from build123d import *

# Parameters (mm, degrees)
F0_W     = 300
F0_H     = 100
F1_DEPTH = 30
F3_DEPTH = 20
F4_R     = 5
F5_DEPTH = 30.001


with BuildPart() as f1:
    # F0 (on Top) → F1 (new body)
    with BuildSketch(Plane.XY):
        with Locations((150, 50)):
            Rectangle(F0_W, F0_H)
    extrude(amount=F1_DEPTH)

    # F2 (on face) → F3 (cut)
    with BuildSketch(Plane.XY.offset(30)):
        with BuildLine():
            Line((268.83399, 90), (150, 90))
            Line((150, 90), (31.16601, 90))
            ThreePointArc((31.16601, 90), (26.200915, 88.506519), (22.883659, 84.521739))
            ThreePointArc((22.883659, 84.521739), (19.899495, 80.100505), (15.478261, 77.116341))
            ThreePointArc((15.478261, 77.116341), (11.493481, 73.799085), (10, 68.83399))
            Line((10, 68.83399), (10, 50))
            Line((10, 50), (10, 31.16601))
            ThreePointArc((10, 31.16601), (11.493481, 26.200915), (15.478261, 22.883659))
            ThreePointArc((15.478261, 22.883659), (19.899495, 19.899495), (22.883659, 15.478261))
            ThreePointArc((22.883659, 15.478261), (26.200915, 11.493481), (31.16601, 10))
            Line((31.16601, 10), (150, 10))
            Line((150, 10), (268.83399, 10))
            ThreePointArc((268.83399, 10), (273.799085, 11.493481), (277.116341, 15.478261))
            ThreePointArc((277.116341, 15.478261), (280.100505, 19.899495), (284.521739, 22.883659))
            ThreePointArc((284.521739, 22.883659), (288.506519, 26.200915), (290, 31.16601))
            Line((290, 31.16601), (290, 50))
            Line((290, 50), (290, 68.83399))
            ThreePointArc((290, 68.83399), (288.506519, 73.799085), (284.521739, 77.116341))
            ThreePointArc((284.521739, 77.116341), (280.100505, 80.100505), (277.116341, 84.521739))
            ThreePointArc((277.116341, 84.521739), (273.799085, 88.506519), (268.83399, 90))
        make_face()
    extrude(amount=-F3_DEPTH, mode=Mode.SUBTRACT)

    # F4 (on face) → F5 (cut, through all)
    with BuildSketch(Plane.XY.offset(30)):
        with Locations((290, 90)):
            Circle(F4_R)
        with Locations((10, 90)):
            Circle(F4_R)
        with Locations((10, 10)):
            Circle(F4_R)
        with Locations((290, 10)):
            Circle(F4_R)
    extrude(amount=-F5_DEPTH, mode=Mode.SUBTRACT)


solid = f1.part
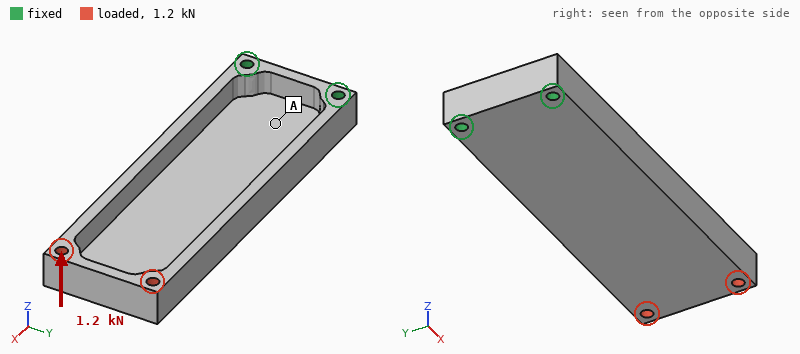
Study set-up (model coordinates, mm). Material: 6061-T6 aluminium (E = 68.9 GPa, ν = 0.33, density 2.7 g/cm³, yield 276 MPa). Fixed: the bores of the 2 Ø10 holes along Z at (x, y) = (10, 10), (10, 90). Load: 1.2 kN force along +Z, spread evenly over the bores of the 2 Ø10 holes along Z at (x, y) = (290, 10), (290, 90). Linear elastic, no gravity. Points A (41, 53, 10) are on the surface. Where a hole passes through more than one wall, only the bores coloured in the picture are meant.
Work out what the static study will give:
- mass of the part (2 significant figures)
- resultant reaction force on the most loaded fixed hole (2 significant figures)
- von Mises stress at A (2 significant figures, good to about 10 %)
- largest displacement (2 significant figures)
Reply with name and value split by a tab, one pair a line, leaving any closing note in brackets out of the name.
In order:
mass of the part	1.2 kg
resultant reaction force on the most loaded fixed hole	1.8 kN
von Mises stress at A	12 MPa
largest displacement	1.6 mm
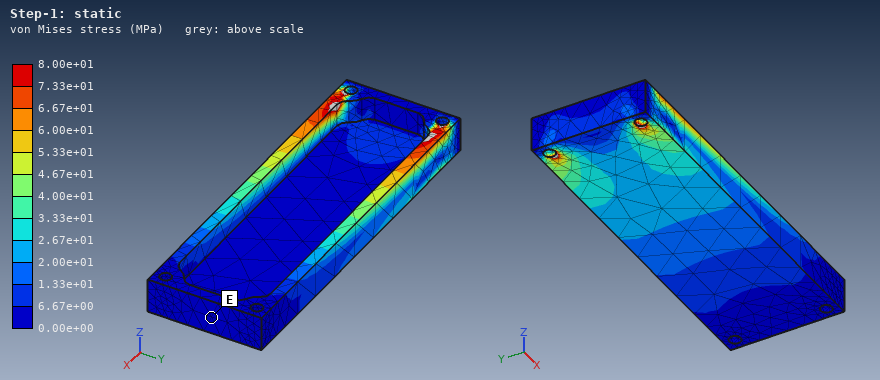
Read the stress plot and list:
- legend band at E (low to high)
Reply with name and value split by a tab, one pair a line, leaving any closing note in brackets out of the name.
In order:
legend band at E	0.00e+00 to 6.67e+00 MPa
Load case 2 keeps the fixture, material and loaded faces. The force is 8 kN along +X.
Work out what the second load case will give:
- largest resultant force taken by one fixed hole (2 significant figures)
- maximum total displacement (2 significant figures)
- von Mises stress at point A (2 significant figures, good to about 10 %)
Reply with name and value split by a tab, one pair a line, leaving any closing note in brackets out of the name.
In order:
largest resultant force taken by one fixed hole	4.0 kN
maximum total displacement	0.31 mm
von Mises stress at point A	4.4 MPa
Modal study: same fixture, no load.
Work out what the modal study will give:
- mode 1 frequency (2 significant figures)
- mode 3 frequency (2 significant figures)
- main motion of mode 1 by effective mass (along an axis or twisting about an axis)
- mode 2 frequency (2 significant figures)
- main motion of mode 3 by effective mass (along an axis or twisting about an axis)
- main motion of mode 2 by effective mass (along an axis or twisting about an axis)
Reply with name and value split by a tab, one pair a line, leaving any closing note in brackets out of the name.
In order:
mode 1 frequency	240 Hz
mode 3 frequency	1000 Hz
main motion of mode 1 by effective mass	along Z
mode 2 frequency	570 Hz
main motion of mode 3 by effective mass	along Y
main motion of mode 2 by effective mass	along Y
